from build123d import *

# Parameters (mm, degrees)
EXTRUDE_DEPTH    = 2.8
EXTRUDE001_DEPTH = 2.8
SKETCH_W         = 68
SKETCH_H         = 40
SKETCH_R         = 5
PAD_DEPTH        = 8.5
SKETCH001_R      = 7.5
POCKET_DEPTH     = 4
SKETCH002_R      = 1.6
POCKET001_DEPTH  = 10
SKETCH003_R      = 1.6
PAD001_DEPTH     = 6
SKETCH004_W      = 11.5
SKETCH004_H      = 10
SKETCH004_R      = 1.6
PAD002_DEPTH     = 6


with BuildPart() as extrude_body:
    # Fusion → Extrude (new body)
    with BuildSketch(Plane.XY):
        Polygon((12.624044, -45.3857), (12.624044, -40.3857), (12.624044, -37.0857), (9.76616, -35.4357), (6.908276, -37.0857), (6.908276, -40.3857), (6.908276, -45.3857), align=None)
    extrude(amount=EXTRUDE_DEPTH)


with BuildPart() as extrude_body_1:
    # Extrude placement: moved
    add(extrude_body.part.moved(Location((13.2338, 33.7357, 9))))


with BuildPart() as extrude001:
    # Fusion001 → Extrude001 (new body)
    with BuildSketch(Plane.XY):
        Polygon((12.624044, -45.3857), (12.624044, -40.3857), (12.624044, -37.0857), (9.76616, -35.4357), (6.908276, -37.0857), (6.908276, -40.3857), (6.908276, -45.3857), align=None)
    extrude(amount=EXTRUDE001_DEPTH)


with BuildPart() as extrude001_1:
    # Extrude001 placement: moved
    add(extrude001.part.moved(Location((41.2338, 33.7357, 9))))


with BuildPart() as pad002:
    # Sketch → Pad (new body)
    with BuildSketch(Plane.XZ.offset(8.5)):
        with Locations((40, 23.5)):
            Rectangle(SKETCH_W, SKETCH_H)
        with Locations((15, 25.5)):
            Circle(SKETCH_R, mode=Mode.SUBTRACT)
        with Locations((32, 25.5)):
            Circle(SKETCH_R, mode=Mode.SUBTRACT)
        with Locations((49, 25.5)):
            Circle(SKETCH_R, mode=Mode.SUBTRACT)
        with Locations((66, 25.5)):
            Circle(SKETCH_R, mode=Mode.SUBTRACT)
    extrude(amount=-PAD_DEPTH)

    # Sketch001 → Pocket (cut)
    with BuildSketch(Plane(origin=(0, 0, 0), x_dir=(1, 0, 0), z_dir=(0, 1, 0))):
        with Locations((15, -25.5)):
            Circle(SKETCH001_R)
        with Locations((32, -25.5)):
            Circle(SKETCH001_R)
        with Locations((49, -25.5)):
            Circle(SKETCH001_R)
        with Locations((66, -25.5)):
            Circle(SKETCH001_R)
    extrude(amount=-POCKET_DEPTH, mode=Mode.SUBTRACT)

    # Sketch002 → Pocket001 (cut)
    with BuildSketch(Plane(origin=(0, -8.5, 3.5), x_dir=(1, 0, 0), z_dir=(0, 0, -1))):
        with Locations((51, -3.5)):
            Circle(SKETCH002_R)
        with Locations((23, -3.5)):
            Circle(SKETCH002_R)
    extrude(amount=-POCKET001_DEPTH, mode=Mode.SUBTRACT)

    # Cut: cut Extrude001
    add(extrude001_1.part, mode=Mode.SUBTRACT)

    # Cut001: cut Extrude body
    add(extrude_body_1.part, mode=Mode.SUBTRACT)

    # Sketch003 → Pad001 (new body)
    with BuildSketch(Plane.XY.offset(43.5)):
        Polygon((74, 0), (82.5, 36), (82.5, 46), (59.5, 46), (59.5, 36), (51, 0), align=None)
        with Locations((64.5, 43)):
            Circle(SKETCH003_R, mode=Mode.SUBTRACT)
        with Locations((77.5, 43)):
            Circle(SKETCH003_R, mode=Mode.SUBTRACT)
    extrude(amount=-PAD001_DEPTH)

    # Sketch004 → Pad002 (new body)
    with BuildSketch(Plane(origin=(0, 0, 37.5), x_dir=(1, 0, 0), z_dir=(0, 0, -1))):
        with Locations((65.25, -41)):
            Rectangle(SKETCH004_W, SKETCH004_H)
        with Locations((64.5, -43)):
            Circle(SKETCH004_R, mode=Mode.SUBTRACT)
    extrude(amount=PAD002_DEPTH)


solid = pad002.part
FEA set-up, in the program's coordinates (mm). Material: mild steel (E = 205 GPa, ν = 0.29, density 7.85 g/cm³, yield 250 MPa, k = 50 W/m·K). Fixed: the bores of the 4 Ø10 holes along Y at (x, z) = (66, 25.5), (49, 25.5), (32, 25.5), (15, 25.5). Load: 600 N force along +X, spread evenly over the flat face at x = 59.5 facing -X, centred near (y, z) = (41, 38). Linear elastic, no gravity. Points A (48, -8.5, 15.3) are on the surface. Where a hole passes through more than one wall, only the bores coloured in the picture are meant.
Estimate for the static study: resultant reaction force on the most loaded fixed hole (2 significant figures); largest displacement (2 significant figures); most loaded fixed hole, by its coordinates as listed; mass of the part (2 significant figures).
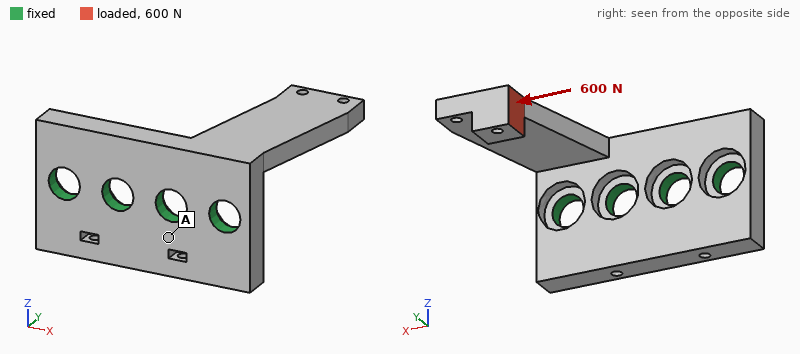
1.3 kN
66 µm
(66, 25.5)
200 g
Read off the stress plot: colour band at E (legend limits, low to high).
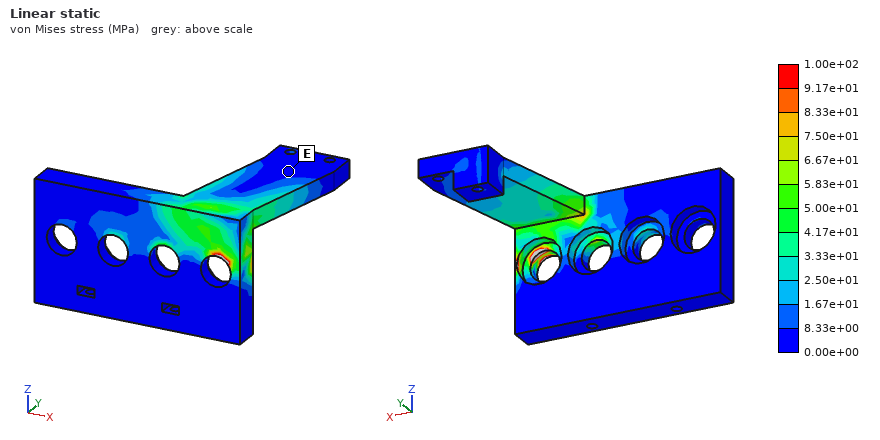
0.00e+00 to 8.33e+00 MPa
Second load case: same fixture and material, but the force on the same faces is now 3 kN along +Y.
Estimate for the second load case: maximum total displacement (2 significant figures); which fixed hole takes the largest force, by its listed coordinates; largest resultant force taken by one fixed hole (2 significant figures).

99 µm
(66, 25.5)
1.8 kN
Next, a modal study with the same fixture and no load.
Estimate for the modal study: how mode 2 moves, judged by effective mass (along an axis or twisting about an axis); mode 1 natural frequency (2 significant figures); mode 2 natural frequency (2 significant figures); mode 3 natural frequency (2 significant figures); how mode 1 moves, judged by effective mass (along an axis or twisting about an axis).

along X
1500 Hz
3500 Hz
7300 Hz
along Z
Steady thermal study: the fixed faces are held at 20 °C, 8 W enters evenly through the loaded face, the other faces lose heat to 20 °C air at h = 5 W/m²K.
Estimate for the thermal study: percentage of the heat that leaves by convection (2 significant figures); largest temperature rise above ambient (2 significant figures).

8.0 %
68 K
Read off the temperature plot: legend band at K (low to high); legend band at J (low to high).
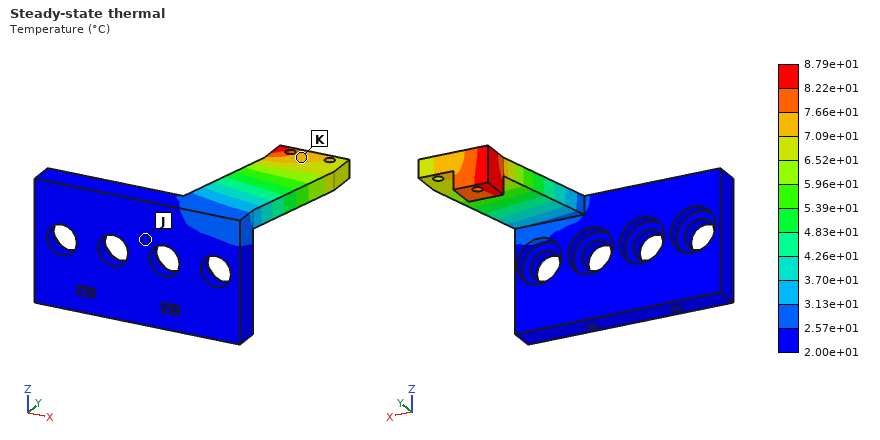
7.09e+01 to 7.66e+01 °C
2.00e+01 to 2.57e+01 °C
